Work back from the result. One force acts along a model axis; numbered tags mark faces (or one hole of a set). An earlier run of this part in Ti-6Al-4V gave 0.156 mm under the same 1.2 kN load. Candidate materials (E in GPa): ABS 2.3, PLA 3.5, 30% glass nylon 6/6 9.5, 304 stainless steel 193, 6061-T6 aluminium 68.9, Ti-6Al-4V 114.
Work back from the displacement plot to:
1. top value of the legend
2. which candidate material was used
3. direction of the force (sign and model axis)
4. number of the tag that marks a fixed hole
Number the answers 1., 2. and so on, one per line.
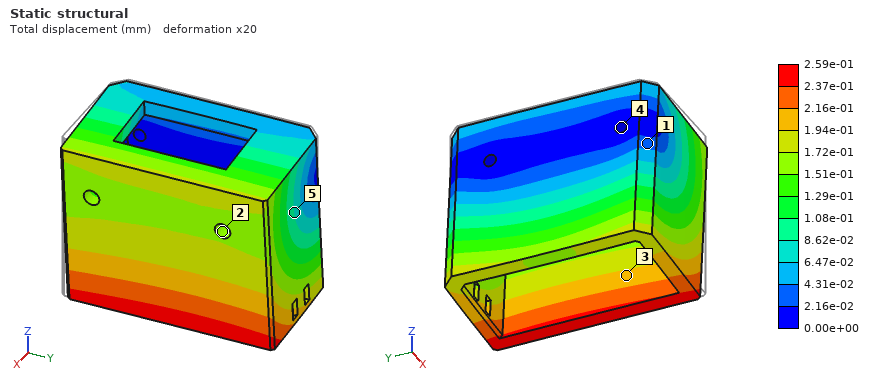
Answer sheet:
1. 2.59e-01 mm
2. 6061-T6 aluminium
3. -Z
4. 4
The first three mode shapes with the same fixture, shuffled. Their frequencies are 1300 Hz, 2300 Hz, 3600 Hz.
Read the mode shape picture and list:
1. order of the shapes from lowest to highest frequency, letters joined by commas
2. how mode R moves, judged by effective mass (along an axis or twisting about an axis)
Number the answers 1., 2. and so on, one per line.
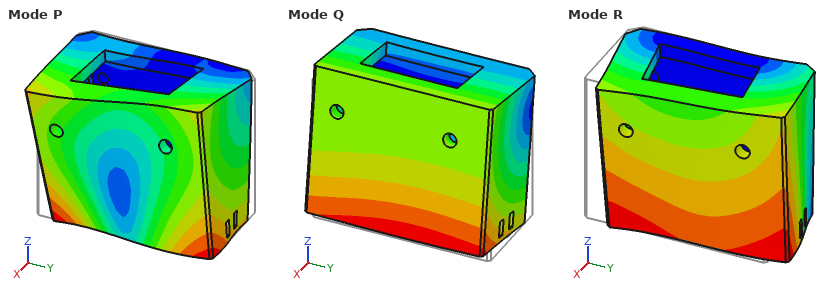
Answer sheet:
1. Q, R, P
2. along Y
